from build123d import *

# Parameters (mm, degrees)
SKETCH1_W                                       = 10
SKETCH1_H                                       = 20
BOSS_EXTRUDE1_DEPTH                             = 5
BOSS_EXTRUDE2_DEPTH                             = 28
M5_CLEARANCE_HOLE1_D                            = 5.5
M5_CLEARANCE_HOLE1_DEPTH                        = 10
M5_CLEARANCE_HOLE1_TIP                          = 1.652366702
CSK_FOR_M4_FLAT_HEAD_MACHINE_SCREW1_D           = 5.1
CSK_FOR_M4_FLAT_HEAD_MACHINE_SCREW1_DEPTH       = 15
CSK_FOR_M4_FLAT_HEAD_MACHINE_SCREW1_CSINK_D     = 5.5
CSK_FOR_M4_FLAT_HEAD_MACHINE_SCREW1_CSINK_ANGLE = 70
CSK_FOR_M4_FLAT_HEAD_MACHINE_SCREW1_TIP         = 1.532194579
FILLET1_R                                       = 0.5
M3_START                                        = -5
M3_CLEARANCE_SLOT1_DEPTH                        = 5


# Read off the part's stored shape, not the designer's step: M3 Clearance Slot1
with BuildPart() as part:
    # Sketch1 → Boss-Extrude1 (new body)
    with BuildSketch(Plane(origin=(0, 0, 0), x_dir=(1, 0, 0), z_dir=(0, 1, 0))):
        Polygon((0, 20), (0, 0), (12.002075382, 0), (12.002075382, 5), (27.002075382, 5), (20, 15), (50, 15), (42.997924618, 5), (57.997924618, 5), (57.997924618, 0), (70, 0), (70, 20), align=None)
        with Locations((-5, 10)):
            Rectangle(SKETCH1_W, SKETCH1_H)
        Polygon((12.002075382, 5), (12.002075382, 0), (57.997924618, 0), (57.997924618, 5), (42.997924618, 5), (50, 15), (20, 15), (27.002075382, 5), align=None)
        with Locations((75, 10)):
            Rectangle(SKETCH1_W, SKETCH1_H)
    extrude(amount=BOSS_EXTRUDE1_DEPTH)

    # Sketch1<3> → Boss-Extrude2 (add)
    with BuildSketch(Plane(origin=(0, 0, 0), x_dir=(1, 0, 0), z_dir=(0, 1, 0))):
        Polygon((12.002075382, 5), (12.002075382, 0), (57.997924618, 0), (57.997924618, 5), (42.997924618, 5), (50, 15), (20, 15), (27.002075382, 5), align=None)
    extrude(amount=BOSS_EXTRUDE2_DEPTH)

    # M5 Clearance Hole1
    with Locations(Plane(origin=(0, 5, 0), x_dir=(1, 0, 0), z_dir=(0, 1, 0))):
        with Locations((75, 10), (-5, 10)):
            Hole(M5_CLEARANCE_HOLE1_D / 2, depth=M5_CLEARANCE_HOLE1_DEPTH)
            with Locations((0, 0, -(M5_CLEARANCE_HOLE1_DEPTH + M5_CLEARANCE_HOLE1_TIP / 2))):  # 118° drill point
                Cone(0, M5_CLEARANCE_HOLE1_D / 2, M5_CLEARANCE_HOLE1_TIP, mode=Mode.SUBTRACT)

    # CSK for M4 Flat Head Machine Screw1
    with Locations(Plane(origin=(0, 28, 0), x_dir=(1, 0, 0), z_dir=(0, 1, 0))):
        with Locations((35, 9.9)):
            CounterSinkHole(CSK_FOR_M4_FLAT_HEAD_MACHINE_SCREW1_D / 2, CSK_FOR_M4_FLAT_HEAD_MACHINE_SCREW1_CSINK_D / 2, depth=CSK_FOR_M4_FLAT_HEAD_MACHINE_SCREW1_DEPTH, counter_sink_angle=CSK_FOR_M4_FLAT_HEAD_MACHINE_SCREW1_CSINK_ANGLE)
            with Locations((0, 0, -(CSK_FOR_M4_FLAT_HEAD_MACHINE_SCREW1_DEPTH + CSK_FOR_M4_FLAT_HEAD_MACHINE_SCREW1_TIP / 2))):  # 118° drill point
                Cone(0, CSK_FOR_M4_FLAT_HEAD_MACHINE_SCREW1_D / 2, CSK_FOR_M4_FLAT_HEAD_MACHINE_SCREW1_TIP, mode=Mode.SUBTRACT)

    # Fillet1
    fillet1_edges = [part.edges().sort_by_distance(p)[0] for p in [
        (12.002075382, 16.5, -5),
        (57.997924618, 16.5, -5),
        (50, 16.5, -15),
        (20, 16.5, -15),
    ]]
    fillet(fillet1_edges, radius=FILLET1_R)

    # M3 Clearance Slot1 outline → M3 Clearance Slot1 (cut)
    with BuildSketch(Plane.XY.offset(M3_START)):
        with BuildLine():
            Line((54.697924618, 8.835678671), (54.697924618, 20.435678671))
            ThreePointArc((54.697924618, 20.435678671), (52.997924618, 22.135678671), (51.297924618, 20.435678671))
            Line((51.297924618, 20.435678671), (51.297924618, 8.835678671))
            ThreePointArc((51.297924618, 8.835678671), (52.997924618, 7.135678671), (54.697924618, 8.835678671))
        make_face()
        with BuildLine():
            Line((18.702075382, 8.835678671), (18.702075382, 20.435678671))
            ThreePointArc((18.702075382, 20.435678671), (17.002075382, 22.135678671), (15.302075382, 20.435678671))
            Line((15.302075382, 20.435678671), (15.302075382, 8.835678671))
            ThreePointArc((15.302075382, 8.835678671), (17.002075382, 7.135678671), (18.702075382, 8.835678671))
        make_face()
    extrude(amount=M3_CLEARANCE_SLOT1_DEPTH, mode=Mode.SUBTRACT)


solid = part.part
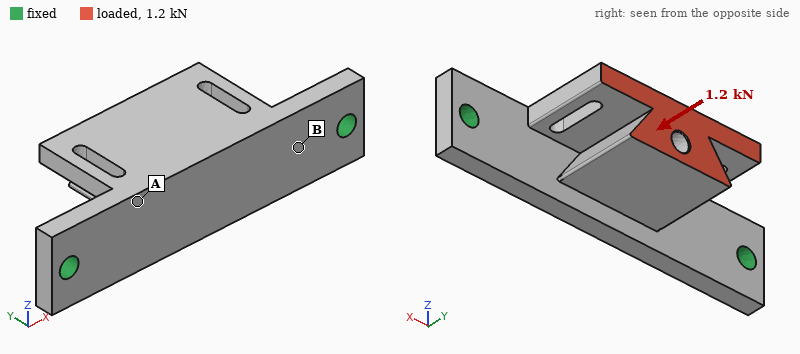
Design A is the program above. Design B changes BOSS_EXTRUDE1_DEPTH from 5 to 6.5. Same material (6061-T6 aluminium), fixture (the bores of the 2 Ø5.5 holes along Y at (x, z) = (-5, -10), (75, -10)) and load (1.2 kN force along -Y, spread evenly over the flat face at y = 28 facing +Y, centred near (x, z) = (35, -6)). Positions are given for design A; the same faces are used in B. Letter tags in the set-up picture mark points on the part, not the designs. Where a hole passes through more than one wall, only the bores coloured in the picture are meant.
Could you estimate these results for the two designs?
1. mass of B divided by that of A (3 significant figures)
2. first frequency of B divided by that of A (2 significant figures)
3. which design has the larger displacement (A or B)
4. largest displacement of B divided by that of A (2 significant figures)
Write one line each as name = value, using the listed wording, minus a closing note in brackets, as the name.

mass of B divided by that of A = 1.10
first frequency of B divided by that of A = 1.4
which design has the larger displacement = A
largest displacement of B divided by that of A = 0.62
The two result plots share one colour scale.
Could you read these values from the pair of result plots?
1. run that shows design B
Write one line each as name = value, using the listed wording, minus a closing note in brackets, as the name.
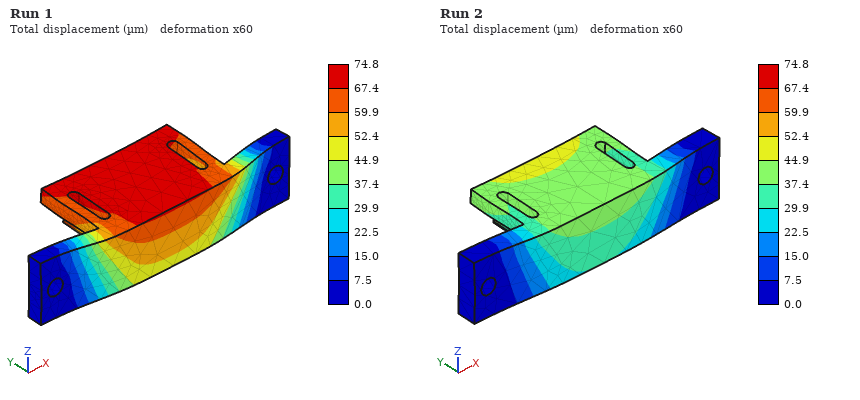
run that shows design B = Run 2
